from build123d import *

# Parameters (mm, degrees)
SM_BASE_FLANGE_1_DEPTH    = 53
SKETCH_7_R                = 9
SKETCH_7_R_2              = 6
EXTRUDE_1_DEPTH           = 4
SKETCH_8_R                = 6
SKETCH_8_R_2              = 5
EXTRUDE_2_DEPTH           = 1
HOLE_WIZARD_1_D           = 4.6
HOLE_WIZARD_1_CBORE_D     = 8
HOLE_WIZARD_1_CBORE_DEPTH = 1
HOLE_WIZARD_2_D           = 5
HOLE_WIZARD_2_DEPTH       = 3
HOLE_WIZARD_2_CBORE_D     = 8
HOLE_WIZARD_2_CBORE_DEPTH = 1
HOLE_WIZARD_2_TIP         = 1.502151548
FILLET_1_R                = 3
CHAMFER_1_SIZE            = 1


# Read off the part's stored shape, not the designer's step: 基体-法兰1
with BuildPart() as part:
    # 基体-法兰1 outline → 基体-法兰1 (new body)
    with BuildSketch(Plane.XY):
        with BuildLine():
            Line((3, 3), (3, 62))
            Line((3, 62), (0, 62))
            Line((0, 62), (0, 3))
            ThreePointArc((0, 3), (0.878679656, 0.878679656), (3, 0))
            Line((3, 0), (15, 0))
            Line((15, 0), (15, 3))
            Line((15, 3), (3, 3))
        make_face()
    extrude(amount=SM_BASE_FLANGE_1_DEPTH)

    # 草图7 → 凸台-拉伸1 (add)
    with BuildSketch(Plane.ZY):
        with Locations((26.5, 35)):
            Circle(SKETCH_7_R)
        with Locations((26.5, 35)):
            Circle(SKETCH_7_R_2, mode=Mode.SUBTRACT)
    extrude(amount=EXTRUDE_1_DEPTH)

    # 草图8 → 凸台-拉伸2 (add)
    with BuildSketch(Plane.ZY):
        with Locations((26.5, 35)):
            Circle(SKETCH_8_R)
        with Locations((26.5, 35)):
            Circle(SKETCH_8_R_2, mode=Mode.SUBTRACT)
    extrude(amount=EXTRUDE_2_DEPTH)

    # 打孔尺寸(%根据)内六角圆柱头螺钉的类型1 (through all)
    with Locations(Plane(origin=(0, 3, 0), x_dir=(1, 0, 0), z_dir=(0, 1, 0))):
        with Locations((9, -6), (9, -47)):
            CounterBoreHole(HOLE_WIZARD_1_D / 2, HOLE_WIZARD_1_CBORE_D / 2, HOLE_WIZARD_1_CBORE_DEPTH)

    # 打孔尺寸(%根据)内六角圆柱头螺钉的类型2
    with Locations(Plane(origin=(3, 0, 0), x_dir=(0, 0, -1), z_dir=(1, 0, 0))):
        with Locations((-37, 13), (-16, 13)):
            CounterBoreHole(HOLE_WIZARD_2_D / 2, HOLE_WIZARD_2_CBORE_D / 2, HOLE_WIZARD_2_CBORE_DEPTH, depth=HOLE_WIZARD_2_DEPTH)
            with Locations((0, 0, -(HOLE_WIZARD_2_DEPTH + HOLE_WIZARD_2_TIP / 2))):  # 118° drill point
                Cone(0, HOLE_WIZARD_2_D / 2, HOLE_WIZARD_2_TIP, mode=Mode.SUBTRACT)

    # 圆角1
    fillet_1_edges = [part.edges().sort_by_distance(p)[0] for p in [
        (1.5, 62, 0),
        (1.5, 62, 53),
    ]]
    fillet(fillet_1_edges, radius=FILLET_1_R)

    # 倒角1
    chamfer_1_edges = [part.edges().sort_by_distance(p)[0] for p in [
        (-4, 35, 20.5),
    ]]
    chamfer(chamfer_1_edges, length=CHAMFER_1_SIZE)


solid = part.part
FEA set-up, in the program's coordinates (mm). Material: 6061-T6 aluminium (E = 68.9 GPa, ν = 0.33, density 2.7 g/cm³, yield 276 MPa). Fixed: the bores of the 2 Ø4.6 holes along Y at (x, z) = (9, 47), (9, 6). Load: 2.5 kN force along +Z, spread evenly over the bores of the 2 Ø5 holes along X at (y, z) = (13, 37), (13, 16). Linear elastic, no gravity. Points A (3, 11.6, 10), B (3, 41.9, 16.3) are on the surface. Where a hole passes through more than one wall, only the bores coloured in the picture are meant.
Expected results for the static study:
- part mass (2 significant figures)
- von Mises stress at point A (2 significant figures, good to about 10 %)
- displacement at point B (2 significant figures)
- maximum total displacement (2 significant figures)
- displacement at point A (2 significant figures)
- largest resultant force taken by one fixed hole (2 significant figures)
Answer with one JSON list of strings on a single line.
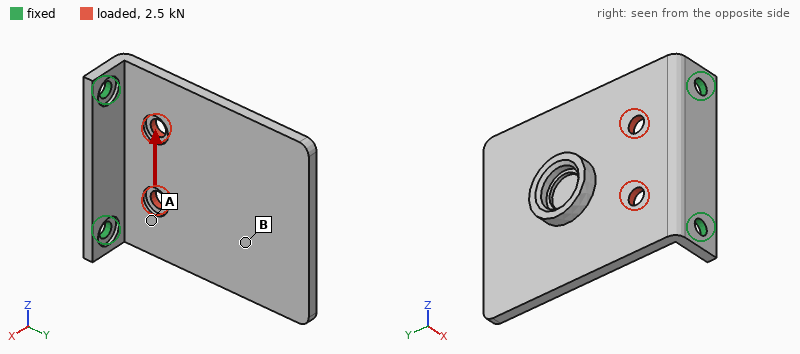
["32 g", "41 MPa", "0.092 mm", "0.15 mm", "0.049 mm", "1.5 kN"]
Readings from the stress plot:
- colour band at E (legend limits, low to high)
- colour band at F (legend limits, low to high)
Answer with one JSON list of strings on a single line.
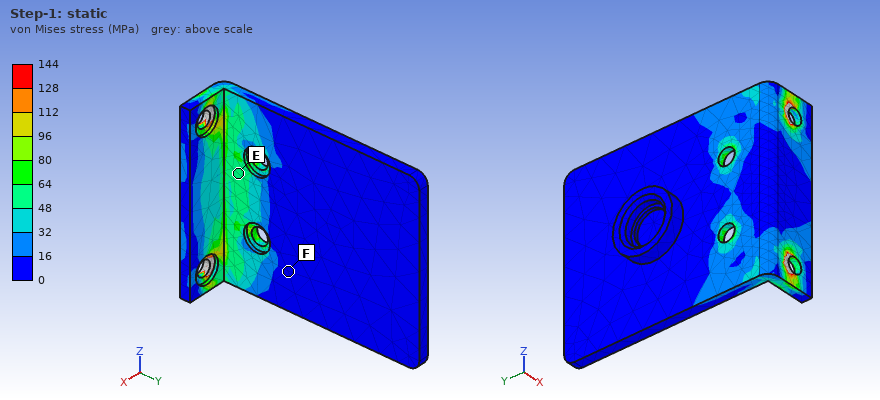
["48 to 64 MPa", "0 to 16 MPa"]
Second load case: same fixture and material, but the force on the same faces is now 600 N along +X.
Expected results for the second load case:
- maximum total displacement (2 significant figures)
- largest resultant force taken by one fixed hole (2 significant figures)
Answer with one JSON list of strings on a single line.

["0.89 mm", "370 N"]
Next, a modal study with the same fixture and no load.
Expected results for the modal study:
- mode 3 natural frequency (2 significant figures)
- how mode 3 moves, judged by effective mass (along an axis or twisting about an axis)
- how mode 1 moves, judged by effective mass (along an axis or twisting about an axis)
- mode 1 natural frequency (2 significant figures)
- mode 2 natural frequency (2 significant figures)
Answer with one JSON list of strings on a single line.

["3200 Hz", "along Z", "along X", "480 Hz", "1700 Hz"]
